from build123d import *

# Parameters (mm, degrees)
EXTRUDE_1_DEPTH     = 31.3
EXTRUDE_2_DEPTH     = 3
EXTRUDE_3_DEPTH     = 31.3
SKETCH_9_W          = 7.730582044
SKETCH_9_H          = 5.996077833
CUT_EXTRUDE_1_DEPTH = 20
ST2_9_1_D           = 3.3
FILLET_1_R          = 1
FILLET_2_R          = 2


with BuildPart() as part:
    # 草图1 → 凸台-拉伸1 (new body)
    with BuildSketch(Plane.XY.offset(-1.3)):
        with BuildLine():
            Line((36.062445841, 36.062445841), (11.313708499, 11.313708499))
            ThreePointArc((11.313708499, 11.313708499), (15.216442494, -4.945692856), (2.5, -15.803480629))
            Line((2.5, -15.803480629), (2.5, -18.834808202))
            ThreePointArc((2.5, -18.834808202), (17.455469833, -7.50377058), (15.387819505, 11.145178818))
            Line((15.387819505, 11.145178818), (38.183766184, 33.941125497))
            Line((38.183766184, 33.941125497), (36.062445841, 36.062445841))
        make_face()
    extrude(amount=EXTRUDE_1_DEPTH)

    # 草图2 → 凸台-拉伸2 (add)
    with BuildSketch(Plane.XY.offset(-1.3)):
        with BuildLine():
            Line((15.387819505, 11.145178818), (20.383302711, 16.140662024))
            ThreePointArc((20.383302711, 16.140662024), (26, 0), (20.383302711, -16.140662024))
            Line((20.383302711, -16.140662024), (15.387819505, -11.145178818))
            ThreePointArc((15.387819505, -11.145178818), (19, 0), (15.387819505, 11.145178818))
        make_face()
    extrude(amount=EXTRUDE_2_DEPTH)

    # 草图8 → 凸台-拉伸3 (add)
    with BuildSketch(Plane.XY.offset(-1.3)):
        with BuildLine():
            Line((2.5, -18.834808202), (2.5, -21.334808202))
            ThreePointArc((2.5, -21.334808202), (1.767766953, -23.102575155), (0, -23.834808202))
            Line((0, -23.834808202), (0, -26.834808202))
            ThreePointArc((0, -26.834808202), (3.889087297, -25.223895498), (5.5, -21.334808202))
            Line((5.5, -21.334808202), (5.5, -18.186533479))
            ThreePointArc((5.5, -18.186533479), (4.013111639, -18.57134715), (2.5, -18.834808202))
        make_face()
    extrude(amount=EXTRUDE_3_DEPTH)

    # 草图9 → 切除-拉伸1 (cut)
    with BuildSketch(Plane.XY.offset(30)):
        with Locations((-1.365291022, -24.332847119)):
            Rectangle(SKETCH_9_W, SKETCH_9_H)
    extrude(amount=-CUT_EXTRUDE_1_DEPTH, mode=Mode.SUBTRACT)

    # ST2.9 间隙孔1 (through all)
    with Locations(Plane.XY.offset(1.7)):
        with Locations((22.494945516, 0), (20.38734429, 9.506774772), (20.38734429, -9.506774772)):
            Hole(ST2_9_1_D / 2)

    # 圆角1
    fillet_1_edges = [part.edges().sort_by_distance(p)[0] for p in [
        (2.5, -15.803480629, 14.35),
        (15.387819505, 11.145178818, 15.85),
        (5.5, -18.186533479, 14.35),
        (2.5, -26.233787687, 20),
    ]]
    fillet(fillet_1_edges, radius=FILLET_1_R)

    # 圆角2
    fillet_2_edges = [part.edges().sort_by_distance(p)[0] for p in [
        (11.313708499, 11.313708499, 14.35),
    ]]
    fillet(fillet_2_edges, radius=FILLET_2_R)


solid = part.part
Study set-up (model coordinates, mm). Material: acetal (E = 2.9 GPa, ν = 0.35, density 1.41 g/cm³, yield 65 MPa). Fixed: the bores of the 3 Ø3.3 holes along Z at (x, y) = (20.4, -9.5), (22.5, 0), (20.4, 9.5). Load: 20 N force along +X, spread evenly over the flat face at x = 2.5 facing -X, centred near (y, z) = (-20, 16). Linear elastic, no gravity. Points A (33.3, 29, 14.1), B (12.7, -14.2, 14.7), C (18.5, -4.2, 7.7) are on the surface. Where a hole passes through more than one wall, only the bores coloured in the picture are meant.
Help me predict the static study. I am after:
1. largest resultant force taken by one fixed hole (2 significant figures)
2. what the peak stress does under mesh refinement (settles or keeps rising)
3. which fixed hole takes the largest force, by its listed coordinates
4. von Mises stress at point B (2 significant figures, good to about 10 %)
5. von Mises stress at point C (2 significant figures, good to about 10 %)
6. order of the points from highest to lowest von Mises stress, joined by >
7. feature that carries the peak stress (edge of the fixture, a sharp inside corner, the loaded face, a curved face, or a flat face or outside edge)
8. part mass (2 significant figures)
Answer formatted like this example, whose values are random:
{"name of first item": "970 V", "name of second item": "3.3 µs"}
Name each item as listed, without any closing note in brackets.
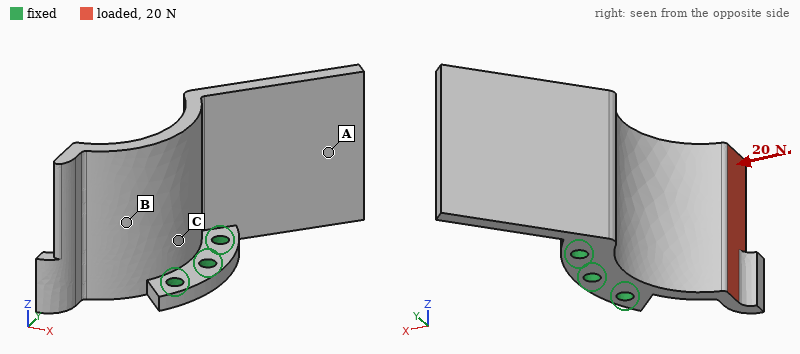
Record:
{"largest resultant force taken by one fixed hole": "30 N", "what the peak stress does under mesh refinement": "keeps rising", "which fixed hole takes the largest force, by its listed coordinates": "(20.4, -9.5)", "von Mises stress at point B": "3.3 MPa", "von Mises stress at point C": "5.4 MPa", "order of the points from highest to lowest von Mises stress, joined by >": "C > B > A", "feature that carries the peak stress": "edge of the fixture", "part mass": "11 g"}
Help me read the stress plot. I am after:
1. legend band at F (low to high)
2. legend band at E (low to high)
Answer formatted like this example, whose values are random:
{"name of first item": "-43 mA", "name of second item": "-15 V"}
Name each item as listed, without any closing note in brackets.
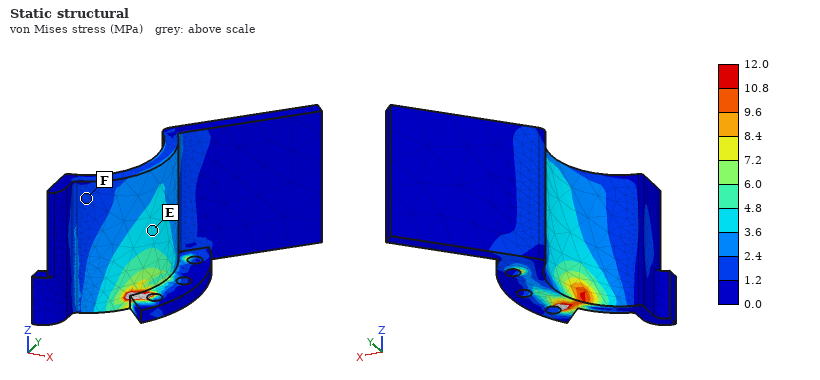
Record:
{"legend band at F": "1.2 to 2.4 MPa", "legend band at E": "3.6 to 4.8 MPa"}
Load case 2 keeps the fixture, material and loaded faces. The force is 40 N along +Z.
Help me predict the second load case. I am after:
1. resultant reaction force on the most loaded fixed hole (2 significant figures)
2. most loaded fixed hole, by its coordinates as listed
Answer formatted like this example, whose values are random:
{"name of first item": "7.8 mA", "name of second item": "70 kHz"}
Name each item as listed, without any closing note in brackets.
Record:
{"resultant reaction force on the most loaded fixed hole": "78 N", "most loaded fixed hole, by its coordinates as listed": "(20.4, -9.5)"}
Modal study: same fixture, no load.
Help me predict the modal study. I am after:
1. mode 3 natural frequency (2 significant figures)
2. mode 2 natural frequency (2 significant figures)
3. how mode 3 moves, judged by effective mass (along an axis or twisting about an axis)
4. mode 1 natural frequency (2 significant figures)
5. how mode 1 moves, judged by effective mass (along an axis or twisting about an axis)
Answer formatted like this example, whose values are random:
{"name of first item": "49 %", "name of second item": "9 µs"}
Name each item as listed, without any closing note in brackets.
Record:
{"mode 3 natural frequency": "820 Hz", "mode 2 natural frequency": "560 Hz", "how mode 3 moves, judged by effective mass": "along Y", "mode 1 natural frequency": "480 Hz", "how mode 1 moves, judged by effective mass": "along X"}
